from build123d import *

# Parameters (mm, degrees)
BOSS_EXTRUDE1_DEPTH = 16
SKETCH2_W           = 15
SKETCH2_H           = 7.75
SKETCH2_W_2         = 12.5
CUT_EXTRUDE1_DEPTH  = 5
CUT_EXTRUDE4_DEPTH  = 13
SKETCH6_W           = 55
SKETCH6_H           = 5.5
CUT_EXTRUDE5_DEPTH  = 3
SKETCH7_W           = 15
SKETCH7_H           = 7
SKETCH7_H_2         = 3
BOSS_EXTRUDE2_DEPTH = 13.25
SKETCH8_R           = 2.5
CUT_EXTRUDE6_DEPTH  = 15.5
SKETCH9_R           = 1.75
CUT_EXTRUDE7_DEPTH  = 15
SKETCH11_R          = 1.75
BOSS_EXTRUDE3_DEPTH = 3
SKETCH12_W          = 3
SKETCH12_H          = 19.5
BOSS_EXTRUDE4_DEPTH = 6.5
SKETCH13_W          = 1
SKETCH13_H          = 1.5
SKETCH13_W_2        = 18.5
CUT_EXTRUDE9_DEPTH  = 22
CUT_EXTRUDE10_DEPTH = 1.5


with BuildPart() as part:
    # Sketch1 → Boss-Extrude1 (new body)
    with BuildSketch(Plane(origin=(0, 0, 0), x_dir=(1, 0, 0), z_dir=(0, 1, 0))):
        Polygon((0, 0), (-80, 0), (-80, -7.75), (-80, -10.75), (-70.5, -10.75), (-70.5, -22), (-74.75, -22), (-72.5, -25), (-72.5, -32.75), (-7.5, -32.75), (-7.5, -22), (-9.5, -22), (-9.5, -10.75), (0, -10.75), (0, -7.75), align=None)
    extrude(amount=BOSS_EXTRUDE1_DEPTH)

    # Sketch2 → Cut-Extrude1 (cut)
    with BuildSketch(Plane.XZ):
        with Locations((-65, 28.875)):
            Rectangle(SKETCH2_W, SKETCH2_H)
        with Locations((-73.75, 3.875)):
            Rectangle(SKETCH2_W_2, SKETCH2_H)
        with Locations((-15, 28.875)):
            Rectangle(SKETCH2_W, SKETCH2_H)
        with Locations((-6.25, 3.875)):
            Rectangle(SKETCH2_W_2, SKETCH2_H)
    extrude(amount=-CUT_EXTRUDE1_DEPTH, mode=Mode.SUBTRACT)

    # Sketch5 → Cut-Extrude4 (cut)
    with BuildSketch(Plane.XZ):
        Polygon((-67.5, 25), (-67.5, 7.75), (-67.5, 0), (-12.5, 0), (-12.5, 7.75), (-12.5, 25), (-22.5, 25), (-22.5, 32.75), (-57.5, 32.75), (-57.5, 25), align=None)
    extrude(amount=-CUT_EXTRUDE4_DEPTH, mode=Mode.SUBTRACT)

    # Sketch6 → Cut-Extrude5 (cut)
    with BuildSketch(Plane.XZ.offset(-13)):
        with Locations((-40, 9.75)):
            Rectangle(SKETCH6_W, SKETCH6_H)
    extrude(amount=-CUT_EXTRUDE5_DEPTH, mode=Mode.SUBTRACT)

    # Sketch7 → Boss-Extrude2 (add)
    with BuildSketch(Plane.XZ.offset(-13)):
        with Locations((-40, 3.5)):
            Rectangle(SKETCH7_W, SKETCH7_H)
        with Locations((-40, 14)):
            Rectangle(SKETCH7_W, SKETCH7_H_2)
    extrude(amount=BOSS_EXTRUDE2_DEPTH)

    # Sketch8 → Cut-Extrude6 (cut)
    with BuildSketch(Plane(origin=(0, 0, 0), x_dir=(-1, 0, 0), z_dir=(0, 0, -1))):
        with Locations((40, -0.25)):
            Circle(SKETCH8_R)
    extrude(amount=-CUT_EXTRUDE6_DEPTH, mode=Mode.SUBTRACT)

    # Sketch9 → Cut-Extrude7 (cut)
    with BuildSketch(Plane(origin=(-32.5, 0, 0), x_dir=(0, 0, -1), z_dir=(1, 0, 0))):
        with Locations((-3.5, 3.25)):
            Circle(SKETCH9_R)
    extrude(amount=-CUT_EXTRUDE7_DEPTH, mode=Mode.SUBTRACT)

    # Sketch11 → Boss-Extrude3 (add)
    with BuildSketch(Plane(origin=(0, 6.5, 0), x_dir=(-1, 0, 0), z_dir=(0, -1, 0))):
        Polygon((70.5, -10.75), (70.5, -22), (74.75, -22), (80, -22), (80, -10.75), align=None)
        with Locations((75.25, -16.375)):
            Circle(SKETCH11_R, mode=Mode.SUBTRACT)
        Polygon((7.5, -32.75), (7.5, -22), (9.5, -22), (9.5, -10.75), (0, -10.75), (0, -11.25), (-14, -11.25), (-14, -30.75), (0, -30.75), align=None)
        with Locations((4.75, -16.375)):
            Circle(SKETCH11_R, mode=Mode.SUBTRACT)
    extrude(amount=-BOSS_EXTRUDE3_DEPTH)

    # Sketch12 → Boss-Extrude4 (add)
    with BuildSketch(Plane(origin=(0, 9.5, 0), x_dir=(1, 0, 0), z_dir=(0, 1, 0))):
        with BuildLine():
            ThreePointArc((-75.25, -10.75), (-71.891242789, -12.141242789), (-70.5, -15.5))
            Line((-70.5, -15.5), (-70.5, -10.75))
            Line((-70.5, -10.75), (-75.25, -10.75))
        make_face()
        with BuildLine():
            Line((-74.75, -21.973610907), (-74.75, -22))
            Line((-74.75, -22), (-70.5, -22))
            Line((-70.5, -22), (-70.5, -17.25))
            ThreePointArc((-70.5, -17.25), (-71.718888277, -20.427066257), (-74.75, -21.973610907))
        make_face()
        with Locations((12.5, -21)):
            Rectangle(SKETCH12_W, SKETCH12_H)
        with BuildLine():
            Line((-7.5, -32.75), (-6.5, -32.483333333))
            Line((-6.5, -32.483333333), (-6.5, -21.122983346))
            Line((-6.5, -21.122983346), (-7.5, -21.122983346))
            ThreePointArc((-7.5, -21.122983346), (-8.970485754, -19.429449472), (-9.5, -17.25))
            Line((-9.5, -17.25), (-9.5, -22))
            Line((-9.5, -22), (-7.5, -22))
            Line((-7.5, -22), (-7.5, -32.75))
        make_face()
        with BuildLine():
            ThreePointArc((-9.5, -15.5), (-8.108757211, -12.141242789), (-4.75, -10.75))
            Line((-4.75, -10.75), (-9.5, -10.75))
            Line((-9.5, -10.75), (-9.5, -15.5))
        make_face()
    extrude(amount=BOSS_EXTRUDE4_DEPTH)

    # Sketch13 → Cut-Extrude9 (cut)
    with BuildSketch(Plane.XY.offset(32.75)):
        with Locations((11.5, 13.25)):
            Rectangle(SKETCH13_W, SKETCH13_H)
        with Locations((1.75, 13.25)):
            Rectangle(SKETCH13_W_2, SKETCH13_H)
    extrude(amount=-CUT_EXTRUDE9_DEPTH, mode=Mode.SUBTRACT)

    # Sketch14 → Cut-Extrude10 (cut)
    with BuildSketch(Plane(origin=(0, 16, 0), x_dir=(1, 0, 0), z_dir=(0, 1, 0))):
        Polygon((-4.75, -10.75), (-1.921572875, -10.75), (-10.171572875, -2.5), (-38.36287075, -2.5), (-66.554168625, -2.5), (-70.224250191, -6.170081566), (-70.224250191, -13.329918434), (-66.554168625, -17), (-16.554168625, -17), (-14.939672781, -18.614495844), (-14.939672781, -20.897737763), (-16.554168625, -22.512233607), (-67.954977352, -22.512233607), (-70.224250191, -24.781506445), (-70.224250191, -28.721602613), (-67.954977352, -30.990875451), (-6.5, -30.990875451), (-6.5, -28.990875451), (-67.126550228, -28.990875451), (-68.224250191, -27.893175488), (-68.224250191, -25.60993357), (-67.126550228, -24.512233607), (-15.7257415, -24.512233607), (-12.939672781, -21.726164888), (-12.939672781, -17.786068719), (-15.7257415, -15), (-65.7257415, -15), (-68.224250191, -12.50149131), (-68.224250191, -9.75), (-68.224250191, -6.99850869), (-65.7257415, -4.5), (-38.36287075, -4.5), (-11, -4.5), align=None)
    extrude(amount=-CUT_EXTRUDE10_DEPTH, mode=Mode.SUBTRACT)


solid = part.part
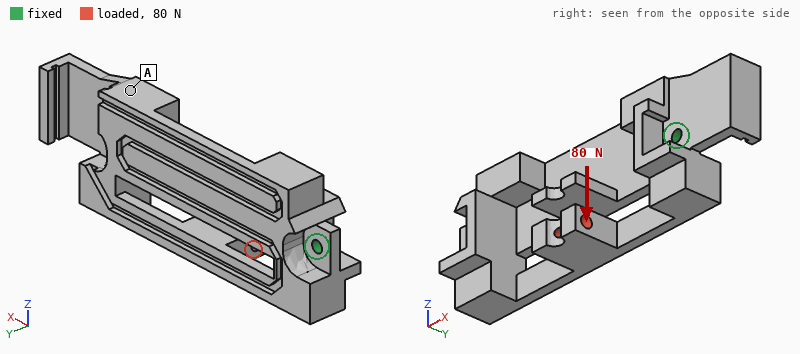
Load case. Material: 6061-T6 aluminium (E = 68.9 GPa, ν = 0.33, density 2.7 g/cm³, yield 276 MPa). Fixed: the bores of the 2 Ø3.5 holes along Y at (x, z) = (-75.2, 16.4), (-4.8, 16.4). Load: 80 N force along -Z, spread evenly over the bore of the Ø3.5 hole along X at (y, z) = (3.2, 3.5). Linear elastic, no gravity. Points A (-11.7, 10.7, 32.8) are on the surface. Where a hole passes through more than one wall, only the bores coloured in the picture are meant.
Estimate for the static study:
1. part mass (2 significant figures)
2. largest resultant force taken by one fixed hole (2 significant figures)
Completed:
40 g
41 N
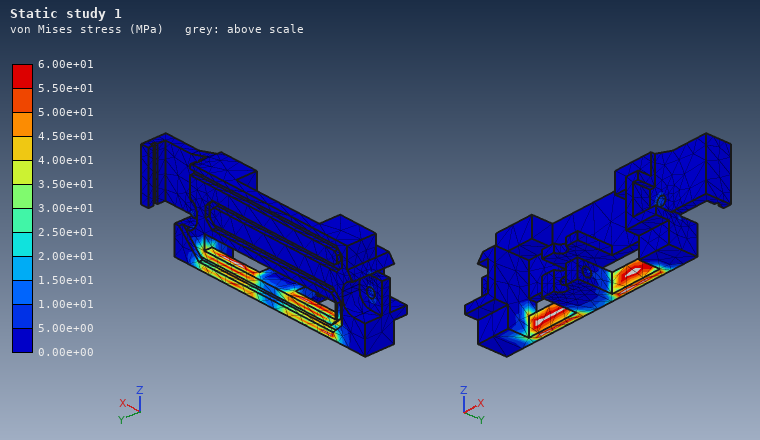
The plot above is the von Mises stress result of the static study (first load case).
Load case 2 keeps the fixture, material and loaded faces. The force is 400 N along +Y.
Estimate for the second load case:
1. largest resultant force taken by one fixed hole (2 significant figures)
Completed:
420 N
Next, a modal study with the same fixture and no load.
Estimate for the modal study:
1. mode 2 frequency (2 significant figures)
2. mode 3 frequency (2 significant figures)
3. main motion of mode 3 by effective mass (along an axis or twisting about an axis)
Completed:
2600 Hz
3900 Hz
along Y
